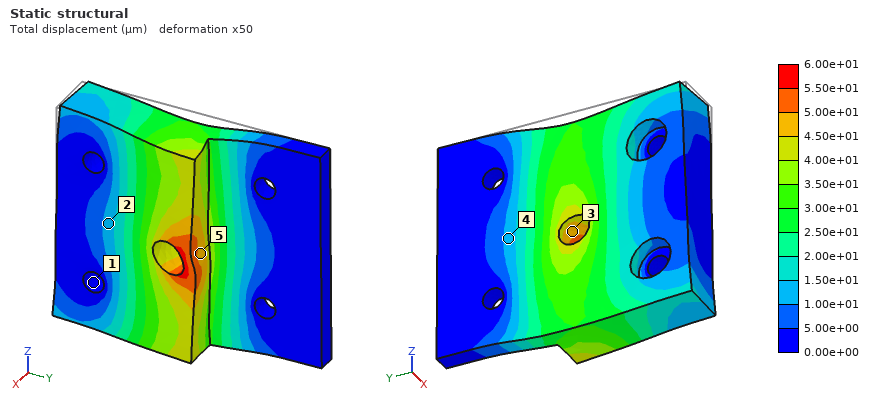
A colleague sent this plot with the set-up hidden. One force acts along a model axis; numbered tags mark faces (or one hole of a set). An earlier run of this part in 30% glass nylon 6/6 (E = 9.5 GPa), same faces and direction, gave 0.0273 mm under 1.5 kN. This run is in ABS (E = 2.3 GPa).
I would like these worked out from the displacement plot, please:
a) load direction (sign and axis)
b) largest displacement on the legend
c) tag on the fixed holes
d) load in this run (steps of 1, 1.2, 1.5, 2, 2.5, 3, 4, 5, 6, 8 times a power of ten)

-Z
6.00e+01 µm
1
800 N
